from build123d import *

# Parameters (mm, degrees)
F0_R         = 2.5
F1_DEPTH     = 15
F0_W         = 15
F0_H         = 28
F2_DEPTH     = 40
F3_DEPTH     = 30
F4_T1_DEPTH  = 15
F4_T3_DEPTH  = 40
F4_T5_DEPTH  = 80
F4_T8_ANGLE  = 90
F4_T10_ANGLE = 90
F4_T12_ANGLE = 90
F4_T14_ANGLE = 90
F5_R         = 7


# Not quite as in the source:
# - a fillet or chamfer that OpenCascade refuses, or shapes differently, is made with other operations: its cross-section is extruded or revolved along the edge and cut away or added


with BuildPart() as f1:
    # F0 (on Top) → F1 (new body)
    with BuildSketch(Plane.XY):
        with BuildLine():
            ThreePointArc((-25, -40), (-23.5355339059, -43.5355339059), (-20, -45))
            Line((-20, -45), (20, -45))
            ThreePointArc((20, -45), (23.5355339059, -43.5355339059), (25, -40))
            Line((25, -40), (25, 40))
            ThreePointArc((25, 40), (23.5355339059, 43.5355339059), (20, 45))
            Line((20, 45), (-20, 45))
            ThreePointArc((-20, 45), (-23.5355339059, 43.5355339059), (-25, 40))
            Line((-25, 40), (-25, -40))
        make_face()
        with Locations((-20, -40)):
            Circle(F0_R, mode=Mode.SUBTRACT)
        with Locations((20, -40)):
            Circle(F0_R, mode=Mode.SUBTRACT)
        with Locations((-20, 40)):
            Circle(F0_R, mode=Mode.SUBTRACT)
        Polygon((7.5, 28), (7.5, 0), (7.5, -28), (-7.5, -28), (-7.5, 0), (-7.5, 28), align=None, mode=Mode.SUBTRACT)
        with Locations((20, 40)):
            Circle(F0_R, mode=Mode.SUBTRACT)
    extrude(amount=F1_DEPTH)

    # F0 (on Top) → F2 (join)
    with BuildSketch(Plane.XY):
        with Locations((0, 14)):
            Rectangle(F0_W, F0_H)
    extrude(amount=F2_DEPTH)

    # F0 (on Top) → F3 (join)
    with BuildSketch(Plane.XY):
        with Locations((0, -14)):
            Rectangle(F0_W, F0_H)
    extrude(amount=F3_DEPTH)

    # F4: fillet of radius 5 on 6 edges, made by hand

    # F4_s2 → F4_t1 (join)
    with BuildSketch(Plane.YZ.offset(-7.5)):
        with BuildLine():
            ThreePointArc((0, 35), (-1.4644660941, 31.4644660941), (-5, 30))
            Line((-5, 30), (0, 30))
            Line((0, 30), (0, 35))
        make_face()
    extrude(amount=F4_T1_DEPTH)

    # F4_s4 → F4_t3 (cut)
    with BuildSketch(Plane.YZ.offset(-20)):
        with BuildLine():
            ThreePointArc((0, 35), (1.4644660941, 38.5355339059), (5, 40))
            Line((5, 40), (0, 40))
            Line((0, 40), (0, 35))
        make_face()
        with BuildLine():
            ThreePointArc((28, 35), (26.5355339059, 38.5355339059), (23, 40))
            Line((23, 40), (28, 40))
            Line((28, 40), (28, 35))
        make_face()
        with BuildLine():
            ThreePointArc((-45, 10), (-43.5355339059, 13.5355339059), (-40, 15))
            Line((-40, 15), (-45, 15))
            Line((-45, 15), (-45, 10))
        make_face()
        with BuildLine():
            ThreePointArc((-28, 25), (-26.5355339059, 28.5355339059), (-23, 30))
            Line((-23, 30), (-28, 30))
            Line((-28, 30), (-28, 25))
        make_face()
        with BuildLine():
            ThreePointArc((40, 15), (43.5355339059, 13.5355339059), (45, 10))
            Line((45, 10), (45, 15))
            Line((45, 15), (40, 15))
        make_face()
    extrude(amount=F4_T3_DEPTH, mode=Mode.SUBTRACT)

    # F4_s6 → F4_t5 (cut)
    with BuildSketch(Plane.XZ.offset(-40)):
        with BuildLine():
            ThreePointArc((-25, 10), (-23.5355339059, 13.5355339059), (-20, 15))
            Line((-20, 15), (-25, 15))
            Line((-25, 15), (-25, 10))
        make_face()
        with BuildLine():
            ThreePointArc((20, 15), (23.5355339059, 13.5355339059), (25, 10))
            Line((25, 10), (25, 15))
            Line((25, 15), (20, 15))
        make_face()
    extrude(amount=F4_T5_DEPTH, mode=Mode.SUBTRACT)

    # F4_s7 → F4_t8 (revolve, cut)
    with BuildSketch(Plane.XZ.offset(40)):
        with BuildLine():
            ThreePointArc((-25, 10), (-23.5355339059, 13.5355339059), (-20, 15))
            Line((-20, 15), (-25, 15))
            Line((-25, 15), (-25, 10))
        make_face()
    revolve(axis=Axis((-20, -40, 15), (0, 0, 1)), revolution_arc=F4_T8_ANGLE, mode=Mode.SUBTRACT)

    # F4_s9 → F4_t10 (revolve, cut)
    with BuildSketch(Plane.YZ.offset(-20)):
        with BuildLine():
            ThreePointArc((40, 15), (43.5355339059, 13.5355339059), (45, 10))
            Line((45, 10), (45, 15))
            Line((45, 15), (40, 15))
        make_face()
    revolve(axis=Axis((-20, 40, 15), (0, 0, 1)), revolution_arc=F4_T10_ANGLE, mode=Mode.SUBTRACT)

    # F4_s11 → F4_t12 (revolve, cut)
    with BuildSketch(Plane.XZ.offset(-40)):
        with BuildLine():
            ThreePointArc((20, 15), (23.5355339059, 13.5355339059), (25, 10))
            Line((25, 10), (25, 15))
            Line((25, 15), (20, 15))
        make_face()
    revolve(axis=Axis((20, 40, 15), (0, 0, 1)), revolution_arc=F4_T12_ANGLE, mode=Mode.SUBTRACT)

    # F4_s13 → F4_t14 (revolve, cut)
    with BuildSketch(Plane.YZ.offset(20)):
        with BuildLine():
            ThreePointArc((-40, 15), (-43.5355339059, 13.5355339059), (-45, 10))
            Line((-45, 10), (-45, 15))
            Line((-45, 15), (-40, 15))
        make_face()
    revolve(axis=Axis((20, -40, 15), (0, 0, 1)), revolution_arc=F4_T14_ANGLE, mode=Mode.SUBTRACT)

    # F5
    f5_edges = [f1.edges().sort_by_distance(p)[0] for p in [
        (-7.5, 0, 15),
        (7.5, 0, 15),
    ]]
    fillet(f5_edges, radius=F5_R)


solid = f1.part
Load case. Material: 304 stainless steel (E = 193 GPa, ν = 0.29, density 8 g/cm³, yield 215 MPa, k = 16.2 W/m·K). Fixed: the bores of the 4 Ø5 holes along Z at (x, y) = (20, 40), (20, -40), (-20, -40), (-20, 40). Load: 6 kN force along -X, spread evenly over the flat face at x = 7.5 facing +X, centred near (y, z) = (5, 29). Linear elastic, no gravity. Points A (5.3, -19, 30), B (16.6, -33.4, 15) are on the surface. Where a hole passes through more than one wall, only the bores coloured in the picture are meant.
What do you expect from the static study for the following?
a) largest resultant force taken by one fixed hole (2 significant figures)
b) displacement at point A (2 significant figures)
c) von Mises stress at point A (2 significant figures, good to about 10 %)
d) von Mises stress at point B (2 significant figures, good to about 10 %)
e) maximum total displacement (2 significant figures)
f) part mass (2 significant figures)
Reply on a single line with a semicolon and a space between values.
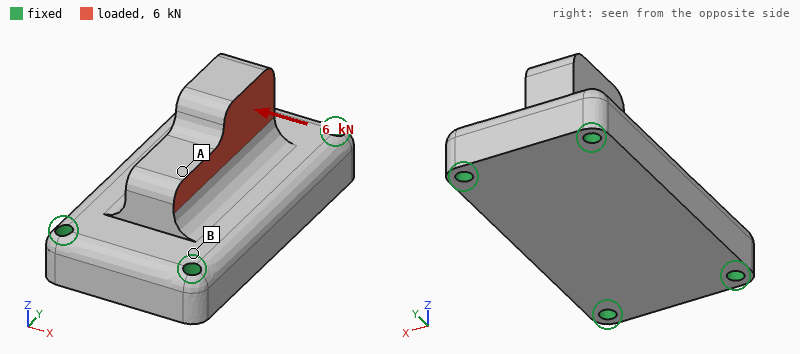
2.8 kN; 7.6 µm; 9.1 MPa; 19 MPa; 18 µm; 660 g
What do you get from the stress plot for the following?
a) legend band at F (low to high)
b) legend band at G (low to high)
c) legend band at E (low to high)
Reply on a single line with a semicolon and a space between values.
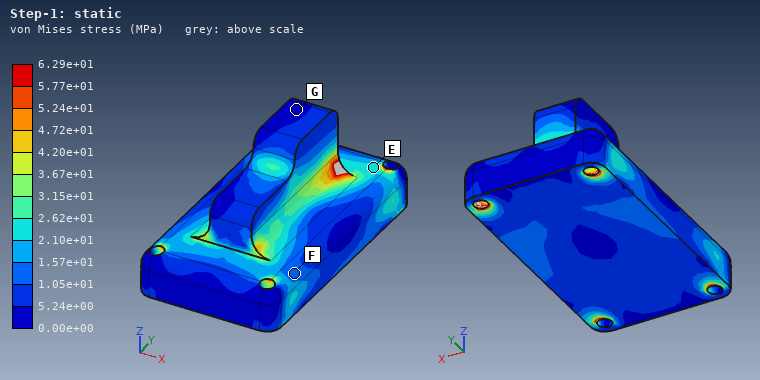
1.05e+01 to 1.57e+01 MPa; 0.00e+00 to 5.24e+00 MPa; 2.10e+01 to 2.62e+01 MPa
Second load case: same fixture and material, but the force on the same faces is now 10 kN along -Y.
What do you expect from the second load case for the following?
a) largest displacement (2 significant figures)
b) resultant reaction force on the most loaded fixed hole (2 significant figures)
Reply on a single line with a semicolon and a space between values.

14 µm; 3.4 kN
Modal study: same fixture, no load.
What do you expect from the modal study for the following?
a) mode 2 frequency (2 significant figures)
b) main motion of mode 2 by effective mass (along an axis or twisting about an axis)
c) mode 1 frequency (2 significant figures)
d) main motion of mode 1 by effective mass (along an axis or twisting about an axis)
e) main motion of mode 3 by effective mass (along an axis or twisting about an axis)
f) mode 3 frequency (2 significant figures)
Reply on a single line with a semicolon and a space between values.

9700 Hz; along X; 8600 Hz; along Z; along X; 15 kHz
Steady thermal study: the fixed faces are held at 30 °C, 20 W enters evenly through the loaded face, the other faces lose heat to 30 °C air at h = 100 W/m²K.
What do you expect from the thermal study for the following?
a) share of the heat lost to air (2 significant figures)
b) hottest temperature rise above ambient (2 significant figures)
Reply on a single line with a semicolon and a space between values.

62 %; 42 K
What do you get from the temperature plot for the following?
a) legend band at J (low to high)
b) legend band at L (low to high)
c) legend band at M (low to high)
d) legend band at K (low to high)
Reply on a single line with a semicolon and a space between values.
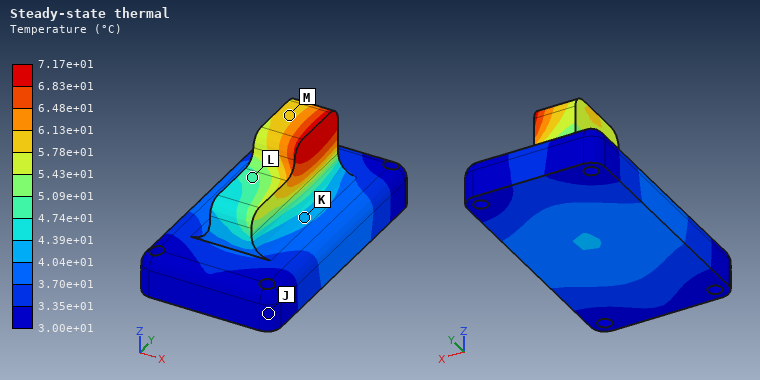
3.00e+01 to 3.35e+01 °C; 4.74e+01 to 5.09e+01 °C; 5.78e+01 to 6.13e+01 °C; 4.04e+01 to 4.39e+01 °C
